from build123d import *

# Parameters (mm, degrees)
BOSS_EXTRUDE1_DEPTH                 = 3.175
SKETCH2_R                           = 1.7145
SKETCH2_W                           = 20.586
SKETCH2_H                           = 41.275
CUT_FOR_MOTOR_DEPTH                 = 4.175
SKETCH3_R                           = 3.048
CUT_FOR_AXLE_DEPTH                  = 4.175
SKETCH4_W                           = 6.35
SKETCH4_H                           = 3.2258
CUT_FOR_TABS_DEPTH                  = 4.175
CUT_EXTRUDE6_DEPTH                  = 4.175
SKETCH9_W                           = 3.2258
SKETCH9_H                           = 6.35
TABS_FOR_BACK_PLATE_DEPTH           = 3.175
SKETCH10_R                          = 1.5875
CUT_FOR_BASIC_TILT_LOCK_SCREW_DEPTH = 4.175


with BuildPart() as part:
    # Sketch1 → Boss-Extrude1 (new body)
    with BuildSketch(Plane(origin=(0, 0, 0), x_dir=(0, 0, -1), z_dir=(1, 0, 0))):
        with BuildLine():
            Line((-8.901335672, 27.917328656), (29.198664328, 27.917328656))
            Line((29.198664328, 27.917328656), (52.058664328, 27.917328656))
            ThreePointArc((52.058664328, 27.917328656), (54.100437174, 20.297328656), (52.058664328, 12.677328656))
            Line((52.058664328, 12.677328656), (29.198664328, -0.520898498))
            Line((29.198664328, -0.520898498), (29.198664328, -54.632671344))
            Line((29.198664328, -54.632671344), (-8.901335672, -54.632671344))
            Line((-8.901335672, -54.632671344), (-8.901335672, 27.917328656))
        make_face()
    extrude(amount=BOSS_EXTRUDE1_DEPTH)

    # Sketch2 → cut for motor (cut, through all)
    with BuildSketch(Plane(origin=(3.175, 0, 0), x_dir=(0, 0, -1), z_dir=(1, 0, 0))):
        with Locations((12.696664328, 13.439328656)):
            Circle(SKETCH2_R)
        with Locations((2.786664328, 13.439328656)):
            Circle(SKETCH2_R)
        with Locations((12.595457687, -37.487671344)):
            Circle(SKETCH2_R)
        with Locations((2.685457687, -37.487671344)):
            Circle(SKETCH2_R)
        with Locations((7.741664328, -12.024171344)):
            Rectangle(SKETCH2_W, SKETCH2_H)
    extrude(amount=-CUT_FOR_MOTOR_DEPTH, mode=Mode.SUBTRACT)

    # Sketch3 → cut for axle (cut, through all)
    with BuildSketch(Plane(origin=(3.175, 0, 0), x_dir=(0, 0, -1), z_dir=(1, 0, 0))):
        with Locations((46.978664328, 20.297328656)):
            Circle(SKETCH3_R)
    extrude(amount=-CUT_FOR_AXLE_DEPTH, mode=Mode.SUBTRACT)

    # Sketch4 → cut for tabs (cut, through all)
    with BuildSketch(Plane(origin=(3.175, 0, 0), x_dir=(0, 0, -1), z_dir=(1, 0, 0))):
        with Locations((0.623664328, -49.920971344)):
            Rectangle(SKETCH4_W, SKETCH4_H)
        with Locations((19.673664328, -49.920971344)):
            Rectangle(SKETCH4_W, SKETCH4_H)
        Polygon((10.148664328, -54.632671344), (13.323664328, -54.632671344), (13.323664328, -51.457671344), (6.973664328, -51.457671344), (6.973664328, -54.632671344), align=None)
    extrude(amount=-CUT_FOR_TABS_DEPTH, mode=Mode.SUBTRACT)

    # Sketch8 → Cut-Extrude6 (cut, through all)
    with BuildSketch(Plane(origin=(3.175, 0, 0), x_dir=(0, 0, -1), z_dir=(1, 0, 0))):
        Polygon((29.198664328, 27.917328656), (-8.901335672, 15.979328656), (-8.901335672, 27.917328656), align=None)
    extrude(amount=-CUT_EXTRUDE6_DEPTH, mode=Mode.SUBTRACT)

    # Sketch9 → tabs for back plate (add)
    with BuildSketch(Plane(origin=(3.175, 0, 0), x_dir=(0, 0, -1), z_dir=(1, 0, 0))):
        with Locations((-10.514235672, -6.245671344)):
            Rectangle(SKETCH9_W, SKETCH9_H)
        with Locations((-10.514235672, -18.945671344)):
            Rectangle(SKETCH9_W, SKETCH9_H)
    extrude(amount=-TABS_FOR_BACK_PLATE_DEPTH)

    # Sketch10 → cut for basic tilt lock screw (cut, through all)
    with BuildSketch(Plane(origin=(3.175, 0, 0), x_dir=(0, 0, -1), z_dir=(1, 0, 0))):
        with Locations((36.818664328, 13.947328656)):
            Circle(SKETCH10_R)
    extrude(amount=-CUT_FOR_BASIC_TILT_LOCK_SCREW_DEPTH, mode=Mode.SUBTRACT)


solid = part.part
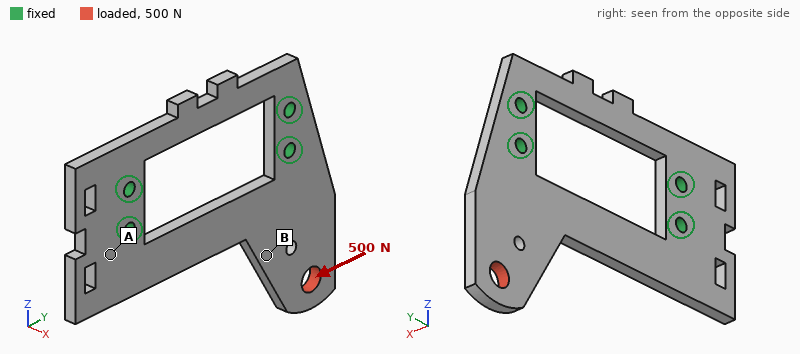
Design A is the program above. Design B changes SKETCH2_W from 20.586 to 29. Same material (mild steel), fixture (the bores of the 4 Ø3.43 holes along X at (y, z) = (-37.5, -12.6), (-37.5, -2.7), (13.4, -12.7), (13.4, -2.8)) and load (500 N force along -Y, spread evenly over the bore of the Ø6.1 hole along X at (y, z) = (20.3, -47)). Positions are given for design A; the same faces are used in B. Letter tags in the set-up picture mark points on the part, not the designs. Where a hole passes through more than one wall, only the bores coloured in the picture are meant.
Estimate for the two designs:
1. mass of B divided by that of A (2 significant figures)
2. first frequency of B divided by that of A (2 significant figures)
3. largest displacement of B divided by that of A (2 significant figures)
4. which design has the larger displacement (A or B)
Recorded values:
0.86
0.96
0.86
A
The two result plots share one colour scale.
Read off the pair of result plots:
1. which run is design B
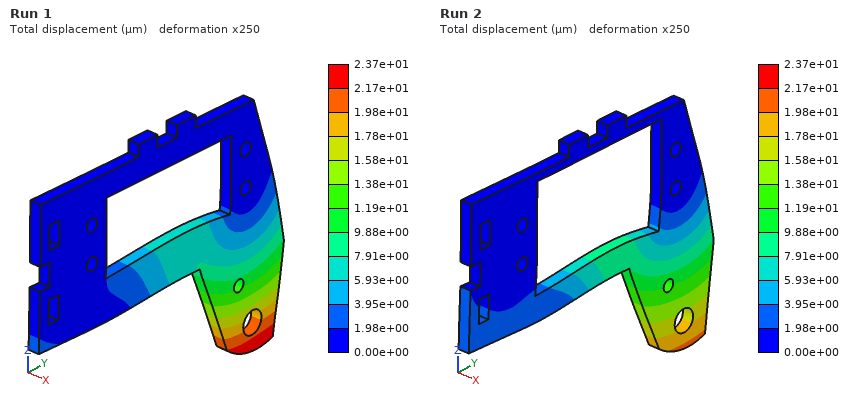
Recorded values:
Run 2
